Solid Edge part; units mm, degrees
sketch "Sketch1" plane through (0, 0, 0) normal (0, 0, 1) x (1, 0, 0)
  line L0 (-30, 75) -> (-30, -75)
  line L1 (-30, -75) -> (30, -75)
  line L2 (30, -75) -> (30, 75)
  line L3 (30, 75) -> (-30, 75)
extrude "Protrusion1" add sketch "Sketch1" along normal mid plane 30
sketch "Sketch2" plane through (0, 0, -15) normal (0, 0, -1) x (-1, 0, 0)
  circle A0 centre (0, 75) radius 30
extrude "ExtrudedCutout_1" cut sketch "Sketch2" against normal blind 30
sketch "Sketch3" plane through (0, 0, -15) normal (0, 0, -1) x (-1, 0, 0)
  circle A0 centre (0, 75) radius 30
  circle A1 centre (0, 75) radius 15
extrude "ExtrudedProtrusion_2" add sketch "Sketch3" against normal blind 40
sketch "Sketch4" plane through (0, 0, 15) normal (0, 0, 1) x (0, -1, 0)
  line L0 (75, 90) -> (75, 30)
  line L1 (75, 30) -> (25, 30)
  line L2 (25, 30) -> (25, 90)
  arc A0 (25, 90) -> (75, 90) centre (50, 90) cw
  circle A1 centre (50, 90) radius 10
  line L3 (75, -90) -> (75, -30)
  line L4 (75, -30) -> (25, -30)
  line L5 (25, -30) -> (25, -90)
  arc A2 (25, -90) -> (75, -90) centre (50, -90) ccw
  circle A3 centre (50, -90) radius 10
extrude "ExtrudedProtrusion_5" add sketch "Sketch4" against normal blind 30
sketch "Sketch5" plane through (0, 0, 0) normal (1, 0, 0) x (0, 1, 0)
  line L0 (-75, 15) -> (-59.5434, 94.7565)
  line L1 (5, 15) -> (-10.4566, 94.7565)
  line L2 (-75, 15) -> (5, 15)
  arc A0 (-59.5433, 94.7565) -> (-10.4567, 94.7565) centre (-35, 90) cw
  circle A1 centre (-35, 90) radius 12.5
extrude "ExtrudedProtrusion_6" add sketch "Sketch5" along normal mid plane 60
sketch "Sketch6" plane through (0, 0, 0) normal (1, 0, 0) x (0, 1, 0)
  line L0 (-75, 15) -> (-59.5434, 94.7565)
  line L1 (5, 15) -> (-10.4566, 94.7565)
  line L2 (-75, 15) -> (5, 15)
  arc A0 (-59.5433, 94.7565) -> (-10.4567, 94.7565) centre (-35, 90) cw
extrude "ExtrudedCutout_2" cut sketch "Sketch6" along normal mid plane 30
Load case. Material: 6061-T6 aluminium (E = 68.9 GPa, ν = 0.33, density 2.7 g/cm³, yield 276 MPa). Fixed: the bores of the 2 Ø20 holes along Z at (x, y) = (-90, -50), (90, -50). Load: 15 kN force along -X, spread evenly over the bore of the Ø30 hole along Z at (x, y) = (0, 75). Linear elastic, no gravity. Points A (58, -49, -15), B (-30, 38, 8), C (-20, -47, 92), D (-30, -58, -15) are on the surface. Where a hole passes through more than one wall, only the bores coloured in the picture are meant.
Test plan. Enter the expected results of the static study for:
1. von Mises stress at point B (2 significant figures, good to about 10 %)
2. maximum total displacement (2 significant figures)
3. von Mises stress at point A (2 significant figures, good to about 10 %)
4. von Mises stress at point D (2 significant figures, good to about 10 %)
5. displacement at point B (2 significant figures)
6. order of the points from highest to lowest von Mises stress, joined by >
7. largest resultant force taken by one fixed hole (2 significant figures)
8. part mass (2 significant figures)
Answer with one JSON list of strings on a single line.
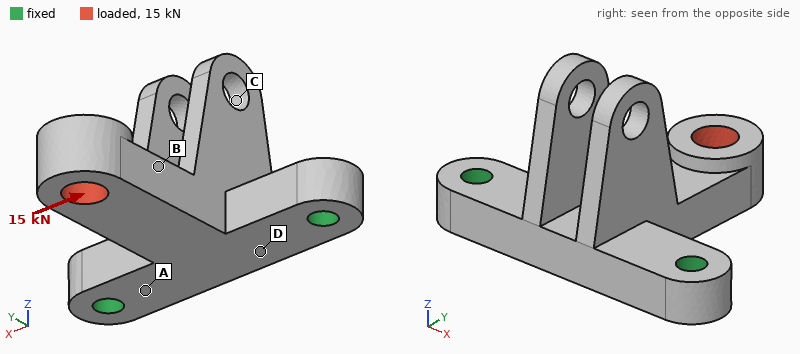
["35 MPa", "0.42 mm", "24 MPa", "15 MPa", "0.20 mm", "B > A > D > C", "15 kN", "1.9 kg"]
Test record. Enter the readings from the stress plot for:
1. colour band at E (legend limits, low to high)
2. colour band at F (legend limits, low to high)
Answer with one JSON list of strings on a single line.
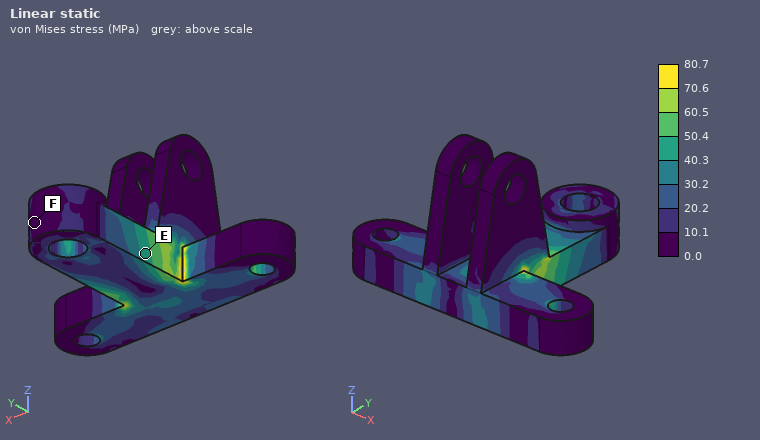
["40.3 to 50.4 MPa", "0.0 to 10.1 MPa"]
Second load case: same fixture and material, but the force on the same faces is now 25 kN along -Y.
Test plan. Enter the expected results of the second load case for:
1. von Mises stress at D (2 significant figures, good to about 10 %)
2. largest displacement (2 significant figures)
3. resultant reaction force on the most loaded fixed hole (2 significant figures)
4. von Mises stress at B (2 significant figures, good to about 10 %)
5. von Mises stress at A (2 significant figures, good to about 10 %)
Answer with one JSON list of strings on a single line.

["9.9 MPa", "0.20 mm", "13 kN", "22 MPa", "14 MPa"]
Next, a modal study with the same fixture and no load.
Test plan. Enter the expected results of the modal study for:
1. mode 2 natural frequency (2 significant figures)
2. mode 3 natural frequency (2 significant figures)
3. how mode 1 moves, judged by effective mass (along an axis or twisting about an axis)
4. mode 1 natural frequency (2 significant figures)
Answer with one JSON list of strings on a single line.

["1500 Hz", "1500 Hz", "along Z", "800 Hz"]
